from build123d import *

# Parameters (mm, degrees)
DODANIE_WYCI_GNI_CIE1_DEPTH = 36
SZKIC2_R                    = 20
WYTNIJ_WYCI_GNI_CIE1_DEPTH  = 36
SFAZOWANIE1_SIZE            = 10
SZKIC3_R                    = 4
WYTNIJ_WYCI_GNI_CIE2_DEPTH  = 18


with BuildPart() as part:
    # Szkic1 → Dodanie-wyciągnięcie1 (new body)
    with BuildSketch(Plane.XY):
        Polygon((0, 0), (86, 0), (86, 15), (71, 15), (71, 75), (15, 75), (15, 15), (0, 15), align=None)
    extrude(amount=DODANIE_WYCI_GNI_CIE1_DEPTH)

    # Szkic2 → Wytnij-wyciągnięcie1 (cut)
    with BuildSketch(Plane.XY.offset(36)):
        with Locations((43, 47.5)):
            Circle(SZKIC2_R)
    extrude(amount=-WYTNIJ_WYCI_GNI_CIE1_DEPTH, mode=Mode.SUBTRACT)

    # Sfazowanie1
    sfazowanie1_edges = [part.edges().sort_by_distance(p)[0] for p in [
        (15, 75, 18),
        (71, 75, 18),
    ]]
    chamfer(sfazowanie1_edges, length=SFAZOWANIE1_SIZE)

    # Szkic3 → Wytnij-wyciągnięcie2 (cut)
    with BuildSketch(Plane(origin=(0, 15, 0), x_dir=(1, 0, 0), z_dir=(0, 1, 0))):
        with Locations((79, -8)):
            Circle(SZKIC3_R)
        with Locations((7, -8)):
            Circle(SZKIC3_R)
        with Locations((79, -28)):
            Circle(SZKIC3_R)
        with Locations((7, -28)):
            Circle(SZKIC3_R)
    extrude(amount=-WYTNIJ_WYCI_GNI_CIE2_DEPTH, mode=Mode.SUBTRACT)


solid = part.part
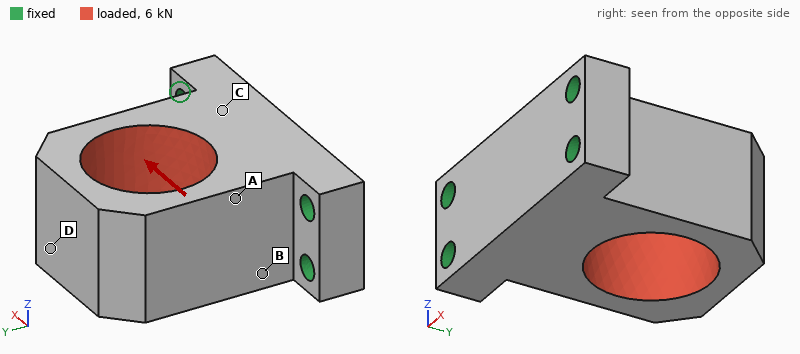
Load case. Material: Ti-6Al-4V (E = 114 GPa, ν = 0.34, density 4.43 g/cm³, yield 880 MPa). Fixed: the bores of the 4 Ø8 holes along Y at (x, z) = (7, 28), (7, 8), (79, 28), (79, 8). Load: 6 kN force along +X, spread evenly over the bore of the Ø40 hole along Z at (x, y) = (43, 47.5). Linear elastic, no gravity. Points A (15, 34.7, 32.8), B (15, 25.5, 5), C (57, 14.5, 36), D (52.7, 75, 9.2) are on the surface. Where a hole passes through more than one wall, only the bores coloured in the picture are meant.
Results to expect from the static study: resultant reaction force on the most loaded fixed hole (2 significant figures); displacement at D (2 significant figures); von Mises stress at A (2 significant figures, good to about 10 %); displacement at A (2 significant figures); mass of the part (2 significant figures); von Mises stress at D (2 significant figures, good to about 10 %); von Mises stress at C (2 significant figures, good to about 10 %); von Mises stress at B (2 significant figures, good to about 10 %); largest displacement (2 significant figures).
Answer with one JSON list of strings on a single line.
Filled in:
["2.5 kN", "33 µm", "27 MPa", "9.1 µm", "510 g", "13 MPa", "8.4 MPa", "23 MPa", "34 µm"]
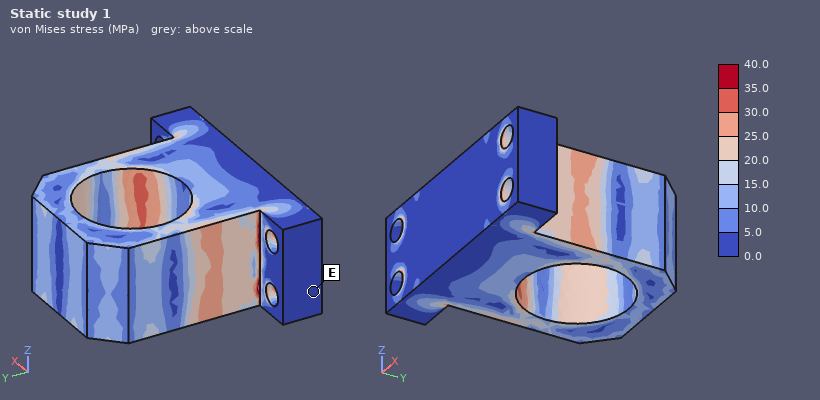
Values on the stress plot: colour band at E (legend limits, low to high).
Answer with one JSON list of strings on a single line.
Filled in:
["0.0 to 5.0 MPa"]
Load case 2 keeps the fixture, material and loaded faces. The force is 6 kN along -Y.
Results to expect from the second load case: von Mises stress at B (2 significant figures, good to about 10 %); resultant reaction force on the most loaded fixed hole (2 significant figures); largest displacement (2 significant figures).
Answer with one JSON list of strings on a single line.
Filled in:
["9.6 MPa", "1.6 kN", "7.9 µm"]
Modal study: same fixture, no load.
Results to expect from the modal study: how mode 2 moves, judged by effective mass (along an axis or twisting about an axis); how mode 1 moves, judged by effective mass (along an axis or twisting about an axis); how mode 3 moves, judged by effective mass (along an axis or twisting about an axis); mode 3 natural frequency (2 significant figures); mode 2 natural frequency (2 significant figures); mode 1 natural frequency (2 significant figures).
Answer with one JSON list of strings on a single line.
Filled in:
["along X", "along Z", "twisting about Y", "7500 Hz", "4600 Hz", "3600 Hz"]
